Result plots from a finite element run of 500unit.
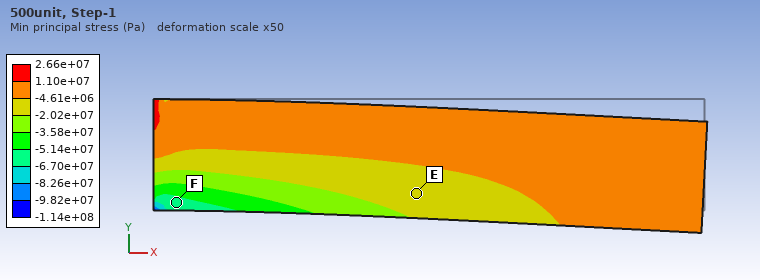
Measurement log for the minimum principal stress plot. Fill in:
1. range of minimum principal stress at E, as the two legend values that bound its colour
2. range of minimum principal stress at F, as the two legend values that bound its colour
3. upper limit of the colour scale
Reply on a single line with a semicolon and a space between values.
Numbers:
-2.02e+07 to -4.61e+06 Pa; -6.70e+07 to -5.14e+07 Pa; 2.66e+07 Pa
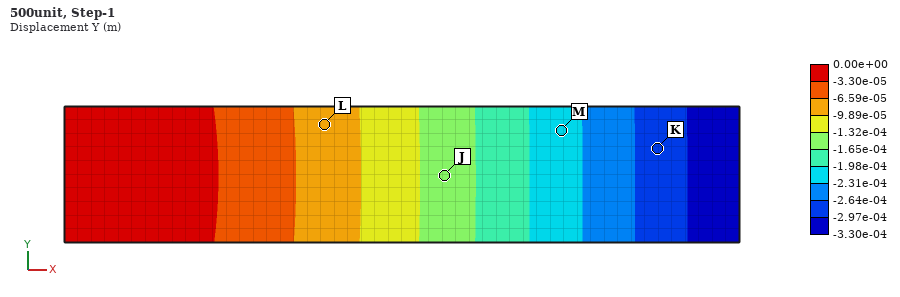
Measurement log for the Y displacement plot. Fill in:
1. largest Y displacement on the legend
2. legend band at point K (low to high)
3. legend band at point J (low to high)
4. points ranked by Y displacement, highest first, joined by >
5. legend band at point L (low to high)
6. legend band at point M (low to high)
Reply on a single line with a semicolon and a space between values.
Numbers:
0.00e+00 m; -2.97e-04 to -2.64e-04 m; -1.65e-04 to -1.32e-04 m; L > J > M > K; -9.89e-05 to -6.59e-05 m; -2.31e-04 to -1.98e-04 m
